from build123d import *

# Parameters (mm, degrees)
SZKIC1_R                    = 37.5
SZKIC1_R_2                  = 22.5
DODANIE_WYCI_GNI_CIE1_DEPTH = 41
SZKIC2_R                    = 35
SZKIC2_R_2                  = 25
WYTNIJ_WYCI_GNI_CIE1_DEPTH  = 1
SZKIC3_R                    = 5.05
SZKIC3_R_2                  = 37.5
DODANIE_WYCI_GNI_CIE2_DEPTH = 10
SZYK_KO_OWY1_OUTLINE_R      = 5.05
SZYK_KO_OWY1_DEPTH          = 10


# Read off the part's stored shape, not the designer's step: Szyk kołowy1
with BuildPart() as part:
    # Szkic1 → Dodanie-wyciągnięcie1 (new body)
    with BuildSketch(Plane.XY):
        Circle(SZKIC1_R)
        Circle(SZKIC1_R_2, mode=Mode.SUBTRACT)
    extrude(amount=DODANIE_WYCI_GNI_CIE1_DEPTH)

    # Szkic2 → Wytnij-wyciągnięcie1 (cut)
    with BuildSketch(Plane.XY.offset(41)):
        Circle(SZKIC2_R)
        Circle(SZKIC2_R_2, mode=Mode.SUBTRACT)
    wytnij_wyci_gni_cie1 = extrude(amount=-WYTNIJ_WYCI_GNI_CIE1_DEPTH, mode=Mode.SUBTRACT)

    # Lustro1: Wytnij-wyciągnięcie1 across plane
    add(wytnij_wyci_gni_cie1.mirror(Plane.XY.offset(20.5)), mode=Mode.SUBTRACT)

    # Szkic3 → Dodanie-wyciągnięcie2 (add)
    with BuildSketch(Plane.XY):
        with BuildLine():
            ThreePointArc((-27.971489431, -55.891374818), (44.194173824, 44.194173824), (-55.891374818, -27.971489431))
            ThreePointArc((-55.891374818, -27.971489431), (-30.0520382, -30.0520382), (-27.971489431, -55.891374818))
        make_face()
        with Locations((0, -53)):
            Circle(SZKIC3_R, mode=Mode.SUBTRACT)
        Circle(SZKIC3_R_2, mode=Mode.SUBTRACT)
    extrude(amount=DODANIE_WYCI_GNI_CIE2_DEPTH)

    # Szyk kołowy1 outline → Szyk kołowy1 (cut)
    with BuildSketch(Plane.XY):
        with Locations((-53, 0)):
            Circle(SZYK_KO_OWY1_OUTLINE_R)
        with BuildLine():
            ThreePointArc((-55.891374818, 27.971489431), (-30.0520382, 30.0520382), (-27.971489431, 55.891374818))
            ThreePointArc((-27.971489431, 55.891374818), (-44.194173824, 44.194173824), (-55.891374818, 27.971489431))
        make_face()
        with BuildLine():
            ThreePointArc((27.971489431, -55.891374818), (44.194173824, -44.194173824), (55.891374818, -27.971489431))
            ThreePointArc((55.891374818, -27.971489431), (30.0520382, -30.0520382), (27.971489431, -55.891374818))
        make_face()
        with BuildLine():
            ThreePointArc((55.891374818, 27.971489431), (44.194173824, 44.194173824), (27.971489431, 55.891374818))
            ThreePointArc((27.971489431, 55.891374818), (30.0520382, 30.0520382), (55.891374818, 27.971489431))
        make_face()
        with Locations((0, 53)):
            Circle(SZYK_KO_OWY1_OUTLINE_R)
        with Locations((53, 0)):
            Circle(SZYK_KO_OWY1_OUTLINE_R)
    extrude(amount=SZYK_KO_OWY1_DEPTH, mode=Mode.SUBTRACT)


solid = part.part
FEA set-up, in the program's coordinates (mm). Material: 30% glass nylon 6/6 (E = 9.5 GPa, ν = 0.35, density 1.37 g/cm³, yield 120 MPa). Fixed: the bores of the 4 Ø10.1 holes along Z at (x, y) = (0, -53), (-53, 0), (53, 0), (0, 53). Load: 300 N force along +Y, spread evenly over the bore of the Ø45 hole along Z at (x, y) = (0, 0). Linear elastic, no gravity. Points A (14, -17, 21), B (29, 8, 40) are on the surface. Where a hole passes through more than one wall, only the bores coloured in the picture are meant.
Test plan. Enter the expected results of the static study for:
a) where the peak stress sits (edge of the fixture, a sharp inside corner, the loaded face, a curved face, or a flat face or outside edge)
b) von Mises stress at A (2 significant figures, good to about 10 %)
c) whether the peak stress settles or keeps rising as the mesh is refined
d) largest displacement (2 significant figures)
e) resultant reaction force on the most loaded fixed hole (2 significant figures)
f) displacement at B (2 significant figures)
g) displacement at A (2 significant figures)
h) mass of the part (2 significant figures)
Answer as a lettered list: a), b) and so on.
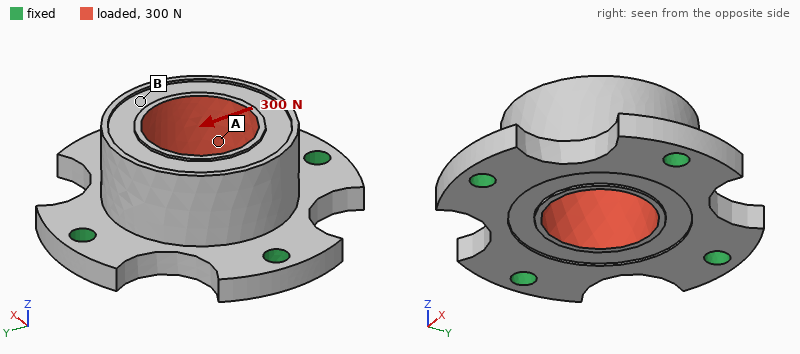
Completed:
a) edge of the fixture
b) 0.18 MPa
c) keeps rising
d) 3.4 µm
e) 120 N
f) 2.7 µm
g) 1.9 µm
h) 220 g
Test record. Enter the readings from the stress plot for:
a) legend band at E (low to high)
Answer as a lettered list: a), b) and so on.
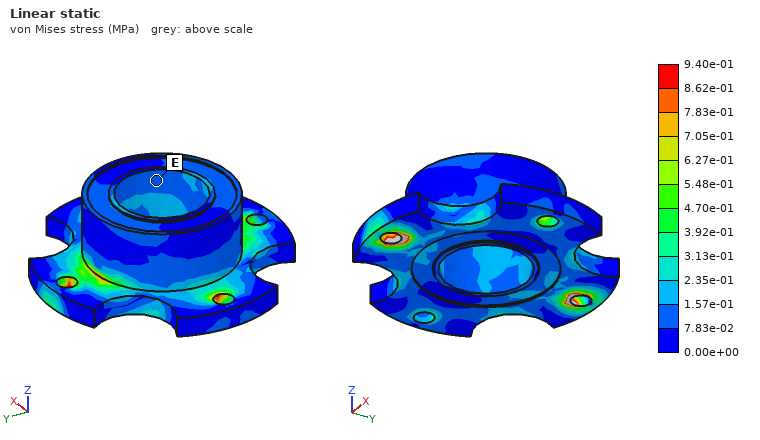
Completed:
a) 7.83e-02 to 1.57e-01 MPa
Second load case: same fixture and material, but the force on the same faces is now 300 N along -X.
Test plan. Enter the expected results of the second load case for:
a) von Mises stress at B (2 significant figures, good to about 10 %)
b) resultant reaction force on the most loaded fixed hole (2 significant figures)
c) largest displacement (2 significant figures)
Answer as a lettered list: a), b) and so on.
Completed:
a) 0.13 MPa
b) 120 N
c) 3.4 µm
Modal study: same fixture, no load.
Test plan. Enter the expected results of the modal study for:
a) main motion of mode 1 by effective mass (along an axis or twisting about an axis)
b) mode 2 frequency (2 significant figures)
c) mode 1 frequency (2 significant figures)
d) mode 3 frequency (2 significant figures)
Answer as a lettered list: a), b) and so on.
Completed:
a) along Z
b) 3900 Hz
c) 3700 Hz
d) 3900 Hz
